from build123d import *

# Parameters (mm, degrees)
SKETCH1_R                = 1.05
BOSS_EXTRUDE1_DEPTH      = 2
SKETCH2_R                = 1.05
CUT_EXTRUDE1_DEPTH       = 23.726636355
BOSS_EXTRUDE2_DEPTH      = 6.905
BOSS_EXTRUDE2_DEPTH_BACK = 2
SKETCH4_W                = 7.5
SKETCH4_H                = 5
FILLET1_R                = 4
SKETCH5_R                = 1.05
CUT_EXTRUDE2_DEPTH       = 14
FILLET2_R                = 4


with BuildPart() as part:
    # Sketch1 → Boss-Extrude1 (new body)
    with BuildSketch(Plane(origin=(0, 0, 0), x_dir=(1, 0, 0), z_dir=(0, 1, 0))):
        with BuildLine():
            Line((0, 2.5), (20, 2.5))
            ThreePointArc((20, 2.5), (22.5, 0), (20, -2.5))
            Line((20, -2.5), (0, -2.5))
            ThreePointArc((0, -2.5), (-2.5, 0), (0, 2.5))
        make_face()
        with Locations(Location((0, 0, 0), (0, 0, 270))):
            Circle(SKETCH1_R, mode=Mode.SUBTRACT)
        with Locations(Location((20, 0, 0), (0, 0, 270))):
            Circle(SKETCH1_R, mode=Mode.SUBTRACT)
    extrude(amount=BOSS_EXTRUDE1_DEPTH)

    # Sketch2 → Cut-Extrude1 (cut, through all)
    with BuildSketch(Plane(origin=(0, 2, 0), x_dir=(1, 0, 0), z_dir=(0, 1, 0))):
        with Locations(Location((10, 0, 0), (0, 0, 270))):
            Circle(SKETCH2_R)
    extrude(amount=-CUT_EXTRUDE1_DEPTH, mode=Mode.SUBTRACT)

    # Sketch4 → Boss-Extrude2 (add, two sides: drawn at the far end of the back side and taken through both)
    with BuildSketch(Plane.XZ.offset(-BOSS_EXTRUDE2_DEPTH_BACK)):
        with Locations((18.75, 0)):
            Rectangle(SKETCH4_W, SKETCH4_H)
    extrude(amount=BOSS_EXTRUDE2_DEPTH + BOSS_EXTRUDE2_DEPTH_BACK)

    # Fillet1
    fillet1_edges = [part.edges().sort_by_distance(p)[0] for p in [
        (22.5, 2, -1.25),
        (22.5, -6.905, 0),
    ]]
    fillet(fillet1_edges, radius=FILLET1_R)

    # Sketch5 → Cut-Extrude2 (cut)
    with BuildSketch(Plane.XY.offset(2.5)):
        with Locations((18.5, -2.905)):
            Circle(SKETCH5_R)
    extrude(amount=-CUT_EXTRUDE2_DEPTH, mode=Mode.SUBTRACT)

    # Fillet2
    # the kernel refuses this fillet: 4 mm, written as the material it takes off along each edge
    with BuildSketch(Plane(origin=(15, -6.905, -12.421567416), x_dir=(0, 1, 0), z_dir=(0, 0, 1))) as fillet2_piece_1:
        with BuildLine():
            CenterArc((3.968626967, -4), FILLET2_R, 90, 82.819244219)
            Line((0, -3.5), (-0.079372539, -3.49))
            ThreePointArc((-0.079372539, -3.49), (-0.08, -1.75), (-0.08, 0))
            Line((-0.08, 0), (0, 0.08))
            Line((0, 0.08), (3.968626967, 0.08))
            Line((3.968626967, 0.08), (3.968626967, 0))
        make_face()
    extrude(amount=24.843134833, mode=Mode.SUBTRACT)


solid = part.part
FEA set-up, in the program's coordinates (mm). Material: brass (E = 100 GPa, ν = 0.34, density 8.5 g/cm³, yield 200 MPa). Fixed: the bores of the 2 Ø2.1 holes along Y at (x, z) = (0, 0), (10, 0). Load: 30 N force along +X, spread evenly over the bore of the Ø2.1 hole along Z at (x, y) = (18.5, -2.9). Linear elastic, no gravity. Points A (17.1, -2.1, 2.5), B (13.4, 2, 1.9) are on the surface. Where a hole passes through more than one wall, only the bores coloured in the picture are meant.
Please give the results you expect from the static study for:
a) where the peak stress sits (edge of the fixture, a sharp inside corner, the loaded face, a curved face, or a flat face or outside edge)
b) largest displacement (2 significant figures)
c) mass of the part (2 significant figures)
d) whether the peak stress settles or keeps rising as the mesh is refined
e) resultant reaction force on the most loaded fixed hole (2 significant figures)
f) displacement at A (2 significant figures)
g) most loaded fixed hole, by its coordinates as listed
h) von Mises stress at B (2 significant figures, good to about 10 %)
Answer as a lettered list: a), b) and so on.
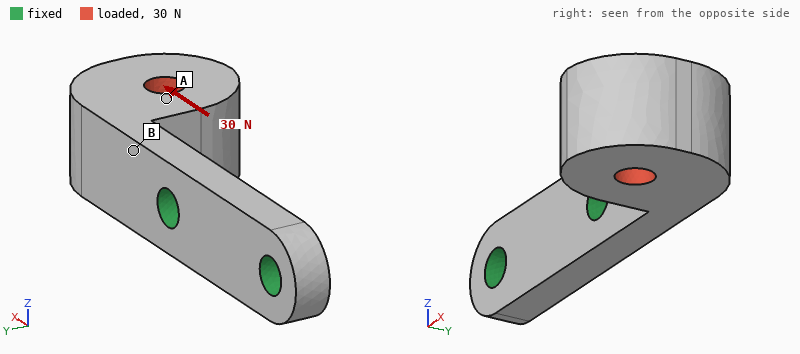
a) edge of the fixture
b) 20 µm
c) 3.6 g
d) keeps rising
e) 29 N
f) 9.2 µm
g) (10, 0)
h) 32 MPa
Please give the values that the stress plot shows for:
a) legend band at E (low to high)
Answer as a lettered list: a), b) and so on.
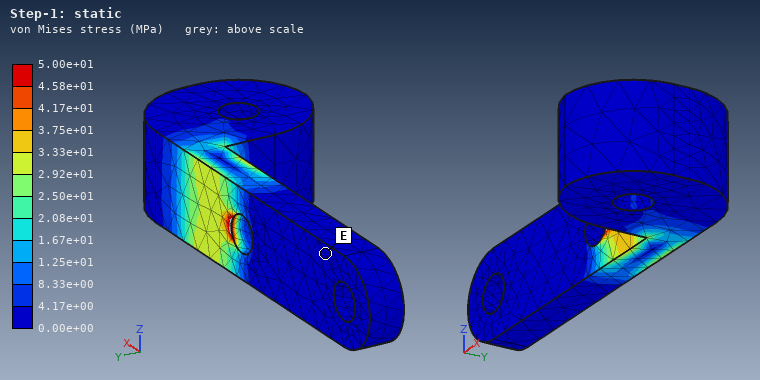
a) 0.00e+00 to 4.17e+00 MPa
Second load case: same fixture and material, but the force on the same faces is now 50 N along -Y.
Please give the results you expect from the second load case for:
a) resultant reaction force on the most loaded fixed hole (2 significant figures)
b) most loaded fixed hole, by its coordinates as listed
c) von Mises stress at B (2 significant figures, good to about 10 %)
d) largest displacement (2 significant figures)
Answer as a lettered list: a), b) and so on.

a) 51 N
b) (10, 0)
c) 75 MPa
d) 46 µm
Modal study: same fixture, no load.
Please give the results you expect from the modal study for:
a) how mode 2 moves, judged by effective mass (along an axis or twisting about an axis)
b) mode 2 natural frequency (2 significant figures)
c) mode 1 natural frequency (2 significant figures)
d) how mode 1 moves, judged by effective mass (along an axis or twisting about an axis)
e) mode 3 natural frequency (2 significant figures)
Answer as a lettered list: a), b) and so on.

a) along Z
b) 6000 Hz
c) 3700 Hz
d) along Y
e) 14 kHz
